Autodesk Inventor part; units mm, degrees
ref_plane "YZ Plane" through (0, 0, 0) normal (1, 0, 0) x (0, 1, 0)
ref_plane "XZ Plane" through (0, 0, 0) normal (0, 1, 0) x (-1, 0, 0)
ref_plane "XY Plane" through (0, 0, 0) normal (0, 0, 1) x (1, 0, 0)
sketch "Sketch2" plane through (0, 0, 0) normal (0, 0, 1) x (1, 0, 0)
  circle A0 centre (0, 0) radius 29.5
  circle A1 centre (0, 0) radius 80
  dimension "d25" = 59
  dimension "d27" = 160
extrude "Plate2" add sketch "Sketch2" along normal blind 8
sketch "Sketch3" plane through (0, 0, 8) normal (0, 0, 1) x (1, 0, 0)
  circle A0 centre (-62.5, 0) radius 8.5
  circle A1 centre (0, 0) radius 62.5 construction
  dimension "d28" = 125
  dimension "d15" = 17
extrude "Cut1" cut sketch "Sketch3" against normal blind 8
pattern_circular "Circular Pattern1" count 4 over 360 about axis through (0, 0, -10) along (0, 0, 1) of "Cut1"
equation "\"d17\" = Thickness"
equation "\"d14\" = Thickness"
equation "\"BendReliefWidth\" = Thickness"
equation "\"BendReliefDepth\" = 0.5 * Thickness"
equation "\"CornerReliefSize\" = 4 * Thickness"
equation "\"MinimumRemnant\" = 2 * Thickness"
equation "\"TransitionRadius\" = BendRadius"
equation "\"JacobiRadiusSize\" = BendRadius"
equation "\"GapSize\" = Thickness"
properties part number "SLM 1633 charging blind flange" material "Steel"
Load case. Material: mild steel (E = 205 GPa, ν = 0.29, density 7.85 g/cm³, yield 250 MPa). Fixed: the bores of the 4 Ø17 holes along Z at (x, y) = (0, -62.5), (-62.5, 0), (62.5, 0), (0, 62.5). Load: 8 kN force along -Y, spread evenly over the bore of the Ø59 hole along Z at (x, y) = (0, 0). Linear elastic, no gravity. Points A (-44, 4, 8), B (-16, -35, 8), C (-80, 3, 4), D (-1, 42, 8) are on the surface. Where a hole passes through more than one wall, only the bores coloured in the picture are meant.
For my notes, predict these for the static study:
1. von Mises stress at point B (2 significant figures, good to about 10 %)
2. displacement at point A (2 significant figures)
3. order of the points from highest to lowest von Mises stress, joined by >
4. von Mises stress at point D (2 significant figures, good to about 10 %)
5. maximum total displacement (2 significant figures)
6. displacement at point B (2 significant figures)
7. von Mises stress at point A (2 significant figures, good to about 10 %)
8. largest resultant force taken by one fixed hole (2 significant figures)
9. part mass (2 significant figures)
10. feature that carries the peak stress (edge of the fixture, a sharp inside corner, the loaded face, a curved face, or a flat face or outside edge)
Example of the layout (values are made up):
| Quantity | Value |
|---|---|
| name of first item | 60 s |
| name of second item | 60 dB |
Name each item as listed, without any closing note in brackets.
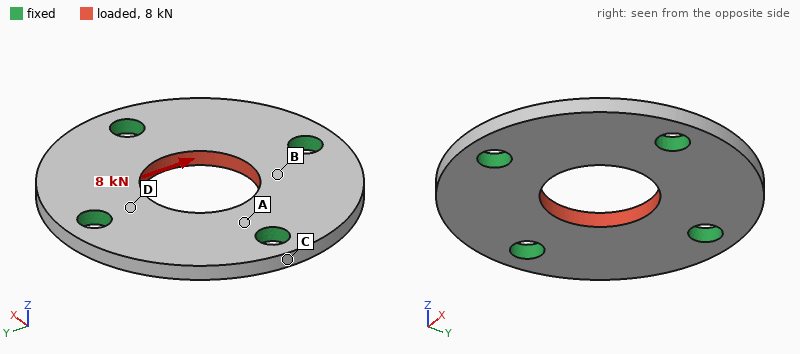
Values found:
| Quantity | Value |
|---|---|
| von Mises stress at point B | 7.0 MPa |
| displacement at point A | 0.67 µm |
| order of the points from highest to lowest von Mises stress, joined by > | D > B > A > C |
| von Mises stress at point D | 8.5 MPa |
| maximum total displacement | 1.6 µm |
| displacement at point B | 1.0 µm |
| von Mises stress at point A | 4.3 MPa |
| largest resultant force taken by one fixed hole | 2.3 kN |
| part mass | 1.0 kg |
| feature that carries the peak stress | edge of the fixture |
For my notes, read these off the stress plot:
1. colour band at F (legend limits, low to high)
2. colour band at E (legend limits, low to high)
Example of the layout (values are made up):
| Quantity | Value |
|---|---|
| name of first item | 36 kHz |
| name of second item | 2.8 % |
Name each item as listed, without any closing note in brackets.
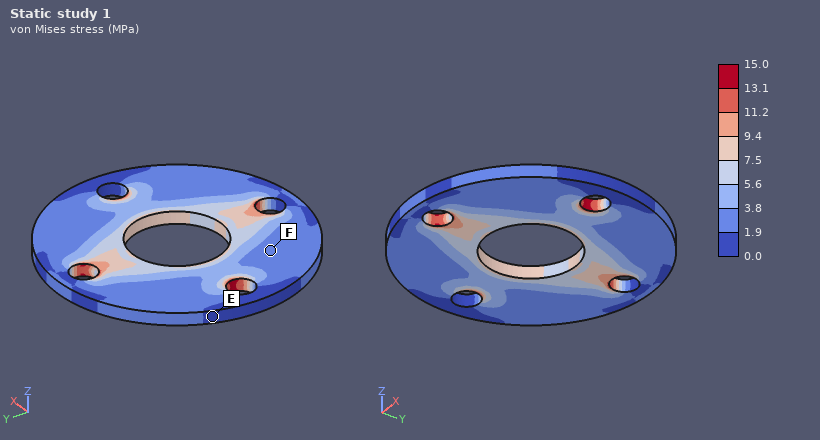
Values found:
| Quantity | Value |
|---|---|
| colour band at F | 1.9 to 3.8 MPa |
| colour band at E | 0.0 to 1.9 MPa |
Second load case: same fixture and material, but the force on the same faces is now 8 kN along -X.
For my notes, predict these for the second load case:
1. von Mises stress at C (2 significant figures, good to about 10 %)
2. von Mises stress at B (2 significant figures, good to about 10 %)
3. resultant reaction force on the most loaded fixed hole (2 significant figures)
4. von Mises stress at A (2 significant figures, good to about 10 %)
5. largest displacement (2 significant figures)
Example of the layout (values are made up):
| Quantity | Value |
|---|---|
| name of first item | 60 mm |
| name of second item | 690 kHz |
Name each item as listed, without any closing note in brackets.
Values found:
| Quantity | Value |
|---|---|
| von Mises stress at C | 2.9 MPa |
| von Mises stress at B | 4.3 MPa |
| resultant reaction force on the most loaded fixed hole | 2.3 kN |
| von Mises stress at A | 8.7 MPa |
| largest displacement | 1.6 µm |
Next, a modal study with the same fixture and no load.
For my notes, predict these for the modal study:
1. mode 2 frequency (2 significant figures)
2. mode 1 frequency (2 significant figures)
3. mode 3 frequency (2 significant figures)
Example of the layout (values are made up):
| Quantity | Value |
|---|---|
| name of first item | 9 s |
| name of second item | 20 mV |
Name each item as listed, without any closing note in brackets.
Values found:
| Quantity | Value |
|---|---|
| mode 2 frequency | 4800 Hz |
| mode 1 frequency | 4700 Hz |
| mode 3 frequency | 4800 Hz |
